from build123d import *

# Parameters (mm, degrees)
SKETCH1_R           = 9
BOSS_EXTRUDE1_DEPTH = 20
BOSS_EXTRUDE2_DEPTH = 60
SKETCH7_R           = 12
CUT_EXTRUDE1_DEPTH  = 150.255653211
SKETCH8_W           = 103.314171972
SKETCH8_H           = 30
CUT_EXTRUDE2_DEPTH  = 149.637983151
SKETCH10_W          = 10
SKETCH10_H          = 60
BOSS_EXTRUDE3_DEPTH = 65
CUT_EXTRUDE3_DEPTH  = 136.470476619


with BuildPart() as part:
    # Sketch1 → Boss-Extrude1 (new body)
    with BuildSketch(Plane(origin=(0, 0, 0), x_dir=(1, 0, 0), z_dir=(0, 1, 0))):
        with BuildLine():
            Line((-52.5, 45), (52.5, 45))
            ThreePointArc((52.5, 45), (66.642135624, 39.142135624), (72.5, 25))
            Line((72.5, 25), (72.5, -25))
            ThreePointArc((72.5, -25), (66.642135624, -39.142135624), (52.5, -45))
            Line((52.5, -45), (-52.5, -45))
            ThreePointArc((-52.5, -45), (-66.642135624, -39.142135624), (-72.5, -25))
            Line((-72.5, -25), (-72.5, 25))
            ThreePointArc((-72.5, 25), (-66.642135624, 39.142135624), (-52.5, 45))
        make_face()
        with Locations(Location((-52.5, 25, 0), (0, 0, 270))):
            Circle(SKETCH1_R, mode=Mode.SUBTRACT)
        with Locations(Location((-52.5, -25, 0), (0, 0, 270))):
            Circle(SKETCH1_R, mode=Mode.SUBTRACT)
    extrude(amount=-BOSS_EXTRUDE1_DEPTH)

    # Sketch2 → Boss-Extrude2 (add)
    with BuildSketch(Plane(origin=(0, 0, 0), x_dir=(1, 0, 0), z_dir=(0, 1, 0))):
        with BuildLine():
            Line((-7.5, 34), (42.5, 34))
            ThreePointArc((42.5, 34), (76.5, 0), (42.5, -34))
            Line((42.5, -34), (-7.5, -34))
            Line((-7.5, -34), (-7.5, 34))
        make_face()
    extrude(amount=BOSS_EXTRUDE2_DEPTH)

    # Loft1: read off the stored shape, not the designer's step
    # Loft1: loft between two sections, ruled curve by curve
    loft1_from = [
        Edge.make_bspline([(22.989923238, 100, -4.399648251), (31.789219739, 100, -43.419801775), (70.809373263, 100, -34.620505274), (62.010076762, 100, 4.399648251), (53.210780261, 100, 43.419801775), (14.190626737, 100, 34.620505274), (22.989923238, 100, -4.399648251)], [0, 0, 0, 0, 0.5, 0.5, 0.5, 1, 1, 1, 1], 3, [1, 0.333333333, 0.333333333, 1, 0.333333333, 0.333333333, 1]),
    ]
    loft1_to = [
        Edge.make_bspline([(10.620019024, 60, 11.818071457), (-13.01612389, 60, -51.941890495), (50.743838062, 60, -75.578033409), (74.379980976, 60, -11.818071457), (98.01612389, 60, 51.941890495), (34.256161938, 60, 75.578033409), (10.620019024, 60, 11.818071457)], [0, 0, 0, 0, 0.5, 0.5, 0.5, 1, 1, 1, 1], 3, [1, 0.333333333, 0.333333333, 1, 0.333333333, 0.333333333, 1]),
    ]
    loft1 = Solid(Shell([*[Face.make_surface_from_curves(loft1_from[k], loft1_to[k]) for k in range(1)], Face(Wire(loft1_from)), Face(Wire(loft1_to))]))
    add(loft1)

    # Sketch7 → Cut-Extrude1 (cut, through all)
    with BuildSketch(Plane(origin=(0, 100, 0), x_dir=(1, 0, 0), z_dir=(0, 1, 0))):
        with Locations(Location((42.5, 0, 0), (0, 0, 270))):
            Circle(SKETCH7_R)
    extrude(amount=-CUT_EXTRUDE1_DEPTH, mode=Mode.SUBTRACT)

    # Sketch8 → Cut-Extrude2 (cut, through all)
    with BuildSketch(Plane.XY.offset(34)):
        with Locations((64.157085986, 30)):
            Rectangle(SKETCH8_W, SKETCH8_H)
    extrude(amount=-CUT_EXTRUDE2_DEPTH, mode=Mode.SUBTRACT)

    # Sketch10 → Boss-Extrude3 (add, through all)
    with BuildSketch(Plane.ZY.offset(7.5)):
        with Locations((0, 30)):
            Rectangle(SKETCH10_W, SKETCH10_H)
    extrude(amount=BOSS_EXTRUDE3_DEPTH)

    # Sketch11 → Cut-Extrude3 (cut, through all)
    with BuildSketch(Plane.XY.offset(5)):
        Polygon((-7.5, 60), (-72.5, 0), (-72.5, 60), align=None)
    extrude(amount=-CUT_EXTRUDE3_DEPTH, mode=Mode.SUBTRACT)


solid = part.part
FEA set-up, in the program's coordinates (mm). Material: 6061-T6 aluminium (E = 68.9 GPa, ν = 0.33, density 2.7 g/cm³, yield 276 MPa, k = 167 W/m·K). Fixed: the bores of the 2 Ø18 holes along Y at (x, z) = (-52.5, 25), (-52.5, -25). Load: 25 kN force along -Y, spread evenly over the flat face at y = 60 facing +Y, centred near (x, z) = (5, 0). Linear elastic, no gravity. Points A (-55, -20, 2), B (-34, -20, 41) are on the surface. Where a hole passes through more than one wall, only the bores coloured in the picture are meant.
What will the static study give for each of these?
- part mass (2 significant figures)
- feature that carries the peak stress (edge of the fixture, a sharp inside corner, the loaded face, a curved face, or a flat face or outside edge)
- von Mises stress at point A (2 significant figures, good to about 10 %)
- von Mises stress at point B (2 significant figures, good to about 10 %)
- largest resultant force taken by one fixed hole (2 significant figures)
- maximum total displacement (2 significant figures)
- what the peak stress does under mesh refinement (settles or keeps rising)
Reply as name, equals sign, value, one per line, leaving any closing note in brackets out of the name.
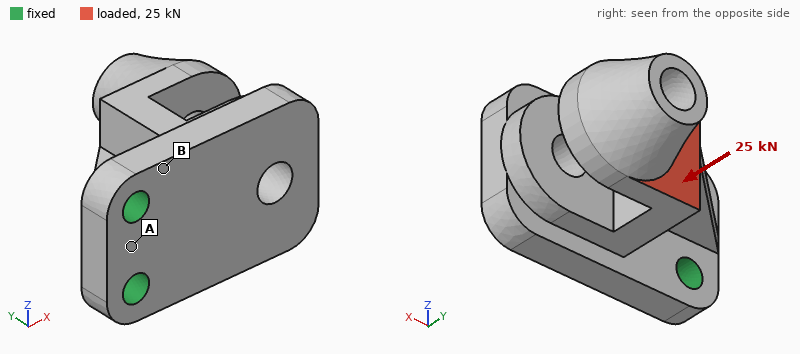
part mass = 1.4 kg
feature that carries the peak stress = edge of the fixture
von Mises stress at point A = 40 MPa
von Mises stress at point B = 100 MPa
largest resultant force taken by one fixed hole = 13 kN
maximum total displacement = 0.76 mm
what the peak stress does under mesh refinement = keeps rising
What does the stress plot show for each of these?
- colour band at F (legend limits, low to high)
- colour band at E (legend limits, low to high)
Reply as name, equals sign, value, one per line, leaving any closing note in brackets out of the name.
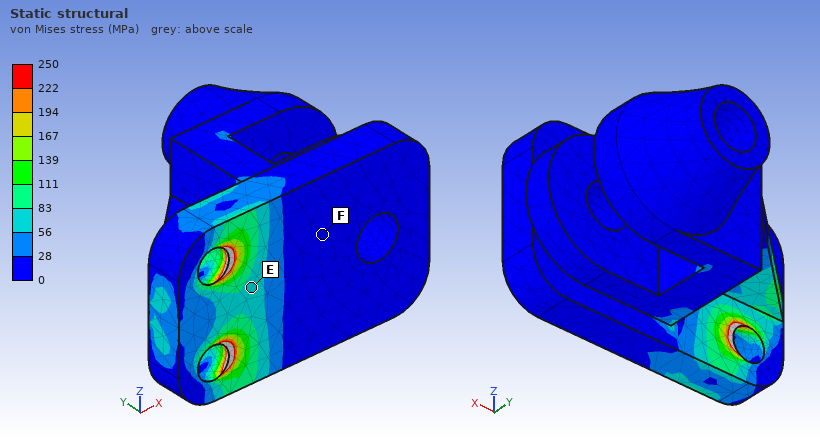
colour band at F = 0 to 28 MPa
colour band at E = 56 to 83 MPa
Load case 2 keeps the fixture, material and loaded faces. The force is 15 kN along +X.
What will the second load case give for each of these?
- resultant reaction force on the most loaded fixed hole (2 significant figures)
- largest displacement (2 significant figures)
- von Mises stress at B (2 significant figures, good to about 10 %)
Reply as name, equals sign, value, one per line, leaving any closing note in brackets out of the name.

resultant reaction force on the most loaded fixed hole = 7.6 kN
largest displacement = 0.85 mm
von Mises stress at B = 81 MPa
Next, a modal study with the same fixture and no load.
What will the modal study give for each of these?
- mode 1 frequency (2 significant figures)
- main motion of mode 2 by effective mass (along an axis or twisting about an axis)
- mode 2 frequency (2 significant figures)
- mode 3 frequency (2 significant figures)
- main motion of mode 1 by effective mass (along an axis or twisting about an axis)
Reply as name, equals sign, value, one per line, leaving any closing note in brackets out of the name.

mode 1 frequency = 790 Hz
main motion of mode 2 by effective mass = along Z
mode 2 frequency = 1200 Hz
mode 3 frequency = 2100 Hz
main motion of mode 1 by effective mass = along Y
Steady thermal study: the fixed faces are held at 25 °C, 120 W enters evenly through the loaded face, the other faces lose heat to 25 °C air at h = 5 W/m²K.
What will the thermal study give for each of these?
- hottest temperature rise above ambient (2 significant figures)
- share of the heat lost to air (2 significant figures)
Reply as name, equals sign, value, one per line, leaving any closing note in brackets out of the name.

hottest temperature rise above ambient = 41 K
share of the heat lost to air = 5.8 %
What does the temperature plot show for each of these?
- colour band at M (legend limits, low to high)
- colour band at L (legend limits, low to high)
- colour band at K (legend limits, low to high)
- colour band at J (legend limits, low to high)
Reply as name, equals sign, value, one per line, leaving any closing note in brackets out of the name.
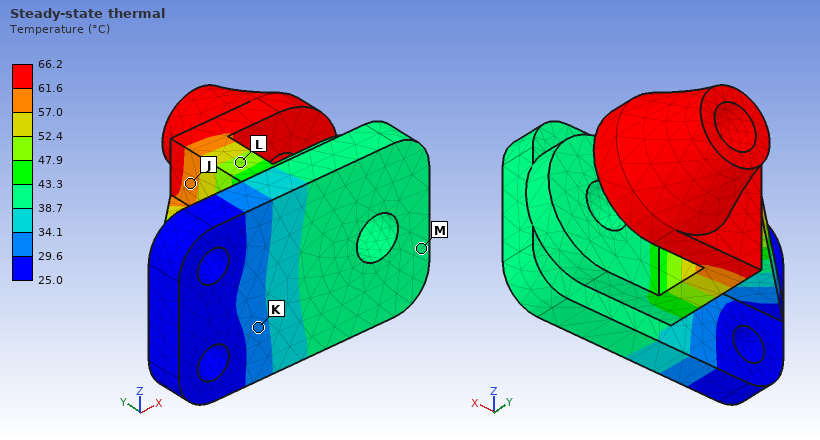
colour band at M = 38.7 to 43.3 °C
colour band at L = 47.9 to 52.4 °C
colour band at K = 29.6 to 34.1 °C
colour band at J = 57.0 to 61.6 °C
